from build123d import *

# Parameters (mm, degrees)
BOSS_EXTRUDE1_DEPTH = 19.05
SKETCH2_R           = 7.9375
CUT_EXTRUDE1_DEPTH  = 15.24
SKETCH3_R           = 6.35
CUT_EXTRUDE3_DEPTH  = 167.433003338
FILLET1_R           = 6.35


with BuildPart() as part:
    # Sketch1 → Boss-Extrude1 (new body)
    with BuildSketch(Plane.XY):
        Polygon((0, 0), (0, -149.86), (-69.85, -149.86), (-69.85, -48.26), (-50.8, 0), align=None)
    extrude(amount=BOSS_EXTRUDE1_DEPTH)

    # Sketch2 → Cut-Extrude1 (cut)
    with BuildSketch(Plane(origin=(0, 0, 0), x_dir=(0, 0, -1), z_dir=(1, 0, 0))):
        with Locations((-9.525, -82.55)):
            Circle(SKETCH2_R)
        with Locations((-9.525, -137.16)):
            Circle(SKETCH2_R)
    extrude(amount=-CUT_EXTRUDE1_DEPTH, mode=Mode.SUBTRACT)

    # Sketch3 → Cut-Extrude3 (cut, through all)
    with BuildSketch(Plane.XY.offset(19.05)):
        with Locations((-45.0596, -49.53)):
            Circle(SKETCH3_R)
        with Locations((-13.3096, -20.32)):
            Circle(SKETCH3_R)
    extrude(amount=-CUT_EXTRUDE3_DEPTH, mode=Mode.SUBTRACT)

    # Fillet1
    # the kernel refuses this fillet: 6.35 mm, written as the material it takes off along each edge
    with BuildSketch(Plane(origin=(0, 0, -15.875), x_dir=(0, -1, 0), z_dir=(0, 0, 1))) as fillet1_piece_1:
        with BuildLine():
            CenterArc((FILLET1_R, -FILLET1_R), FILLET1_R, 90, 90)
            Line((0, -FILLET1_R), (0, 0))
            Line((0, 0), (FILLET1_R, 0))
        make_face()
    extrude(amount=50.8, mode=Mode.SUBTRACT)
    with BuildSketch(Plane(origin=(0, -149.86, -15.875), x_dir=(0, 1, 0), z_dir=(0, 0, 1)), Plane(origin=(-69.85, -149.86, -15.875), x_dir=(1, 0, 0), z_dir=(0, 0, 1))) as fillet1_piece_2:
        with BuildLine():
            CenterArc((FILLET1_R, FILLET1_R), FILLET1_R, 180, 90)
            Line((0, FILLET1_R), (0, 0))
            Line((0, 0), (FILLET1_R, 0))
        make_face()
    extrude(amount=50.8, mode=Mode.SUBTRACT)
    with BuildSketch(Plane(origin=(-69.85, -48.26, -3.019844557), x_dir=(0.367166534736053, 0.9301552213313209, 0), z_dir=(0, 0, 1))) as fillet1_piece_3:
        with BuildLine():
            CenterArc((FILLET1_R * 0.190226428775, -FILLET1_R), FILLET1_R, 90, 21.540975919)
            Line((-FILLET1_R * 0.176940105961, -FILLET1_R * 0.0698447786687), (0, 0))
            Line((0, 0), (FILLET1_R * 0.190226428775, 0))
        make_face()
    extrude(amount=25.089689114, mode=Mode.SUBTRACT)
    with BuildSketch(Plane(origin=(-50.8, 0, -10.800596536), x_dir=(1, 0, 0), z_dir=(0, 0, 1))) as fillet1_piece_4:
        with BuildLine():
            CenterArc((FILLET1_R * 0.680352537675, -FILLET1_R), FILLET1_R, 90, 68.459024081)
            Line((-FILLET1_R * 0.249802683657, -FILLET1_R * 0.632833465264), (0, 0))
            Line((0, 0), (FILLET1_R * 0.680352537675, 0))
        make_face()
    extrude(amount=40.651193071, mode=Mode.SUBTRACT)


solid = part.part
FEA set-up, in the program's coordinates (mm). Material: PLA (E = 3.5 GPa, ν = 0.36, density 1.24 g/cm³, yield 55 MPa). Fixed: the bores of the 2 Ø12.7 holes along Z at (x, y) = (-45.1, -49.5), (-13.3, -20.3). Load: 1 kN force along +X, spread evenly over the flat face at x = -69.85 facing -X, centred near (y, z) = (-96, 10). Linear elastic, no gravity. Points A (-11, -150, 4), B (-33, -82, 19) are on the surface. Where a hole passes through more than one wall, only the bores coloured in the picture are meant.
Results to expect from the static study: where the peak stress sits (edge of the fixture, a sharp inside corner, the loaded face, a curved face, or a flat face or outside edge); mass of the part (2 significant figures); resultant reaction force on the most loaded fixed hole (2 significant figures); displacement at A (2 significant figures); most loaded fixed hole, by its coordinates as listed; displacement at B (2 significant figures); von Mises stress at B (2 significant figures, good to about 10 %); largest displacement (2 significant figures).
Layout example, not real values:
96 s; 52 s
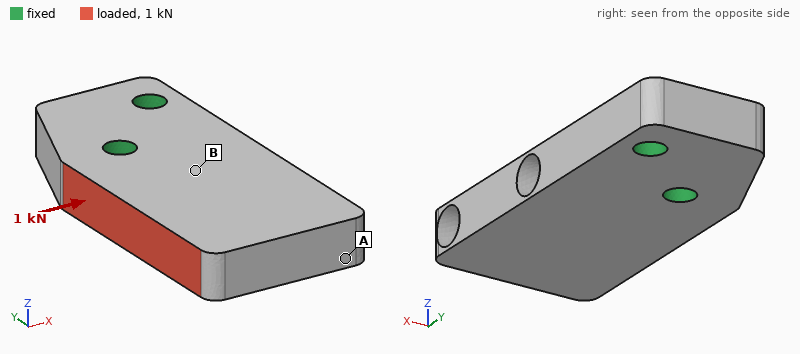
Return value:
a curved face; 220 g; 1.5 kN; 0.18 mm; (-45.1, -49.5); 0.048 mm; 1.6 MPa; 0.18 mm
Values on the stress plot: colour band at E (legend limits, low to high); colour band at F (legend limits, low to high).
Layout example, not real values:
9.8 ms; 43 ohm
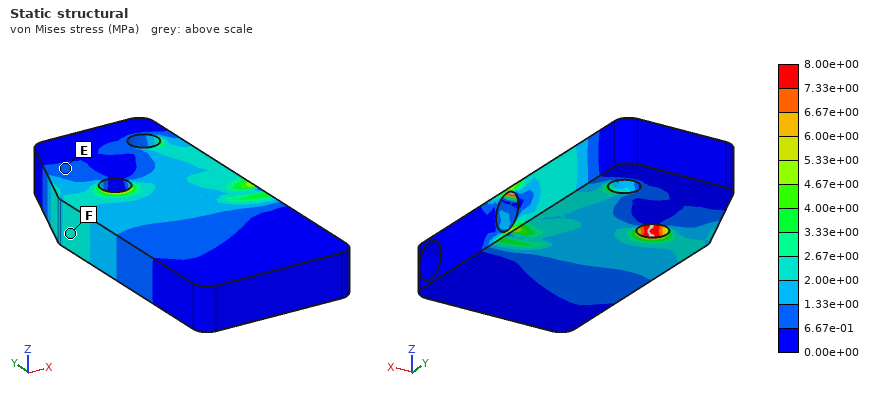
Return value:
6.67e-01 to 1.33e+00 MPa; 2.00e+00 to 2.67e+00 MPa
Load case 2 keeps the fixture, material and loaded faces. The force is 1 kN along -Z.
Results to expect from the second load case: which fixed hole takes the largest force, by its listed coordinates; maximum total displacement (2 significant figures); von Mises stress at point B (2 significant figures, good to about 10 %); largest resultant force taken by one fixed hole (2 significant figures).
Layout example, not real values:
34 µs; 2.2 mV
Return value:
(-45.1, -49.5); 1.1 mm; 6.7 MPa; 1.4 kN
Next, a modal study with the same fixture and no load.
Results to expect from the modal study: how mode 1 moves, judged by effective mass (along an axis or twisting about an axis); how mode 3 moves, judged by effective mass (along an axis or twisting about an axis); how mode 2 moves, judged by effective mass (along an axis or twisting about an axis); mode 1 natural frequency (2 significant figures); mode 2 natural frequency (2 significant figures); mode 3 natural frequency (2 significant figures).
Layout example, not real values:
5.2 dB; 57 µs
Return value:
along Z; twisting about Y; along X; 490 Hz; 1100 Hz; 1300 Hz
